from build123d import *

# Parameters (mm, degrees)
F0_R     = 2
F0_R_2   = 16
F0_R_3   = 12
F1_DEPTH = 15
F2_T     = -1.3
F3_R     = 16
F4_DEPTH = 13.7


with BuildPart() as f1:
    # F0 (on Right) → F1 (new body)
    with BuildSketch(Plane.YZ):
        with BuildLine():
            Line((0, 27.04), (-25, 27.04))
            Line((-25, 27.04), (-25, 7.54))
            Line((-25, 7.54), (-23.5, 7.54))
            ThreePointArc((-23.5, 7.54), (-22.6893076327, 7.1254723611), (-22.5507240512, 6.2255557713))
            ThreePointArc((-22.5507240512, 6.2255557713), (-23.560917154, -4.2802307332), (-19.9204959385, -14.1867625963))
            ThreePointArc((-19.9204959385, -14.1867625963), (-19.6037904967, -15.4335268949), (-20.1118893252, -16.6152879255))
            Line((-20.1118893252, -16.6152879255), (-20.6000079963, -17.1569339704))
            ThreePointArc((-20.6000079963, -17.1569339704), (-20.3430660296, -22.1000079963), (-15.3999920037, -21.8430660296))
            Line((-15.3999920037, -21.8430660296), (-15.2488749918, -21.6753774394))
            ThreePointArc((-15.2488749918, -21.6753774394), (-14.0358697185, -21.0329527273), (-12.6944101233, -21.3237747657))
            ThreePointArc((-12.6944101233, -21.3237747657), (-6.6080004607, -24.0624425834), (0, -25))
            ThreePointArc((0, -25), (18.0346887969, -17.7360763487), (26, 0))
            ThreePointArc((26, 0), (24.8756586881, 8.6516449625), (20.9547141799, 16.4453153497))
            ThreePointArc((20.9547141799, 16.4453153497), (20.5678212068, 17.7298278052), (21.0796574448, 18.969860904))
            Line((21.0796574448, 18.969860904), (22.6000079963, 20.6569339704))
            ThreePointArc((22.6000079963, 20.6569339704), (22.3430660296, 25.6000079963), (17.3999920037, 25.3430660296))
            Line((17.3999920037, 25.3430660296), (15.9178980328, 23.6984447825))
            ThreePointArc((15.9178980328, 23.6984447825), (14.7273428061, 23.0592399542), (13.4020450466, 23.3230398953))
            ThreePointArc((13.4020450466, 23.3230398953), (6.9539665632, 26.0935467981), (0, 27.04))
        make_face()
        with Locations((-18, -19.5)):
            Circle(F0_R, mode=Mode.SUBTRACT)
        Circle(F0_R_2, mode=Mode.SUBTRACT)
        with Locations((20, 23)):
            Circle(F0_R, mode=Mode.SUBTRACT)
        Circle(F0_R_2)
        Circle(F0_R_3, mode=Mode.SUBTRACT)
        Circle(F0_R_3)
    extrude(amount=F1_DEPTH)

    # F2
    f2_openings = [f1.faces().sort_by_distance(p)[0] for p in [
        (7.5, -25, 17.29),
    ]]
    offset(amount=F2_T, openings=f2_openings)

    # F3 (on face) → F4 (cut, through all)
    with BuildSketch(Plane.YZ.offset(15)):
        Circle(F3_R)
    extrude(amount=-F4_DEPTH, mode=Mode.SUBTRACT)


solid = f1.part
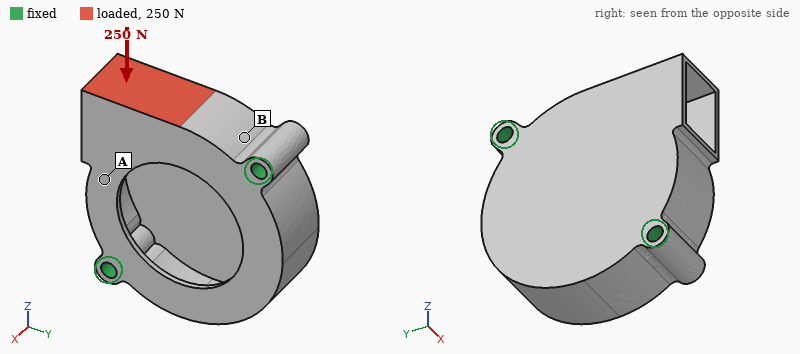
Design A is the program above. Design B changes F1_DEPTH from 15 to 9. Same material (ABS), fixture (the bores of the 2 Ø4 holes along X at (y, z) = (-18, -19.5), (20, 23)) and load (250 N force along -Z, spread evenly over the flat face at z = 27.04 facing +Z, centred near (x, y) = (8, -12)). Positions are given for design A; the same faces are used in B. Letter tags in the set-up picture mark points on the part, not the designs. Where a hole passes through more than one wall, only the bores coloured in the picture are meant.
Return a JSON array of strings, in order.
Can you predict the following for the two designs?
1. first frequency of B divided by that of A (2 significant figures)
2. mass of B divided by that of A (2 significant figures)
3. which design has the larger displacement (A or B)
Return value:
["0.96", "0.82", "A"]
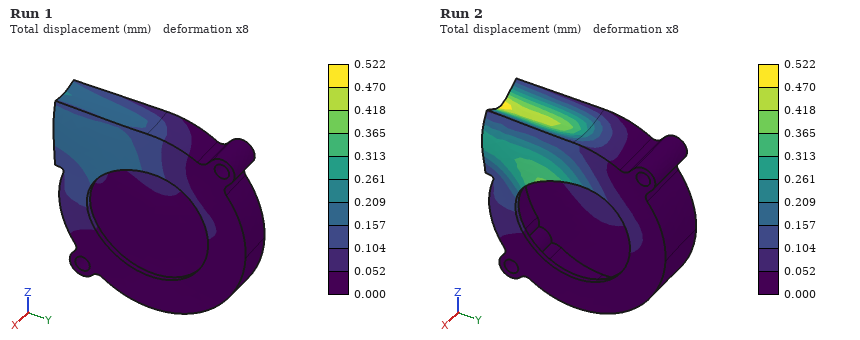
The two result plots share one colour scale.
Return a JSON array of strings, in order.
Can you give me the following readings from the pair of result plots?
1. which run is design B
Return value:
["Run 1"]
